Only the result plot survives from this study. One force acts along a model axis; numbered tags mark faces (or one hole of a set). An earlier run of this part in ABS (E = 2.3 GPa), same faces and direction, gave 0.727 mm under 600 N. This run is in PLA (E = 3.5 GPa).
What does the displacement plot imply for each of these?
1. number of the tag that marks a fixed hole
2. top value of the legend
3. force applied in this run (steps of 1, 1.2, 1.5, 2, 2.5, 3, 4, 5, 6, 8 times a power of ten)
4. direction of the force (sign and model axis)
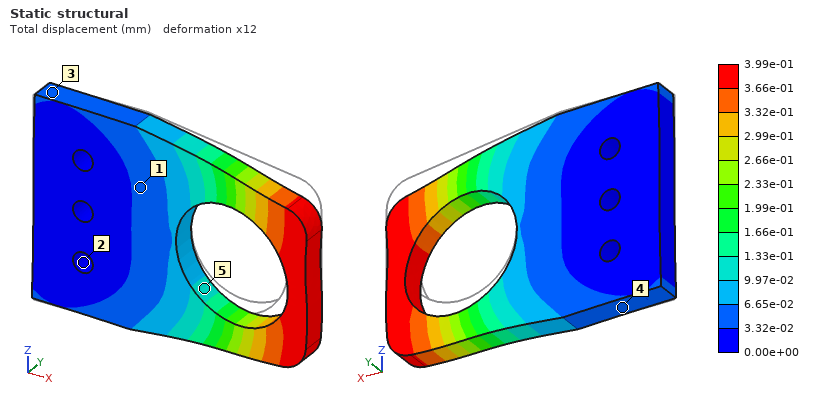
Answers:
2
3.99e-01 mm
500 N
-Z
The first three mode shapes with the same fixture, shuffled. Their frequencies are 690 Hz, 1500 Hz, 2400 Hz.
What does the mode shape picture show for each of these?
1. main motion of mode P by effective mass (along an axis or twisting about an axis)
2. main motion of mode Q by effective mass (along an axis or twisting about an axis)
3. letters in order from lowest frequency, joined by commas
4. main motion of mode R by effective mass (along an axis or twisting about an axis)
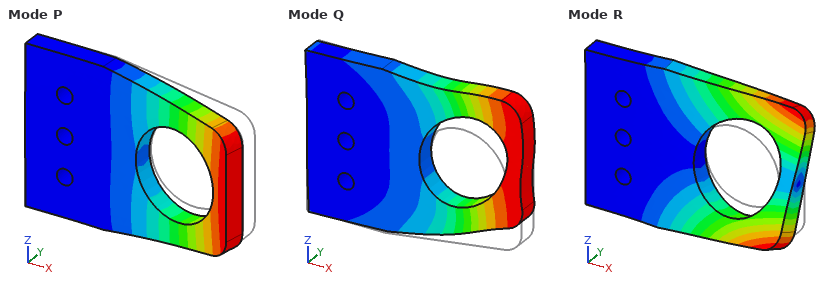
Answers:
along Y
along Z
P, R, Q
twisting about X
